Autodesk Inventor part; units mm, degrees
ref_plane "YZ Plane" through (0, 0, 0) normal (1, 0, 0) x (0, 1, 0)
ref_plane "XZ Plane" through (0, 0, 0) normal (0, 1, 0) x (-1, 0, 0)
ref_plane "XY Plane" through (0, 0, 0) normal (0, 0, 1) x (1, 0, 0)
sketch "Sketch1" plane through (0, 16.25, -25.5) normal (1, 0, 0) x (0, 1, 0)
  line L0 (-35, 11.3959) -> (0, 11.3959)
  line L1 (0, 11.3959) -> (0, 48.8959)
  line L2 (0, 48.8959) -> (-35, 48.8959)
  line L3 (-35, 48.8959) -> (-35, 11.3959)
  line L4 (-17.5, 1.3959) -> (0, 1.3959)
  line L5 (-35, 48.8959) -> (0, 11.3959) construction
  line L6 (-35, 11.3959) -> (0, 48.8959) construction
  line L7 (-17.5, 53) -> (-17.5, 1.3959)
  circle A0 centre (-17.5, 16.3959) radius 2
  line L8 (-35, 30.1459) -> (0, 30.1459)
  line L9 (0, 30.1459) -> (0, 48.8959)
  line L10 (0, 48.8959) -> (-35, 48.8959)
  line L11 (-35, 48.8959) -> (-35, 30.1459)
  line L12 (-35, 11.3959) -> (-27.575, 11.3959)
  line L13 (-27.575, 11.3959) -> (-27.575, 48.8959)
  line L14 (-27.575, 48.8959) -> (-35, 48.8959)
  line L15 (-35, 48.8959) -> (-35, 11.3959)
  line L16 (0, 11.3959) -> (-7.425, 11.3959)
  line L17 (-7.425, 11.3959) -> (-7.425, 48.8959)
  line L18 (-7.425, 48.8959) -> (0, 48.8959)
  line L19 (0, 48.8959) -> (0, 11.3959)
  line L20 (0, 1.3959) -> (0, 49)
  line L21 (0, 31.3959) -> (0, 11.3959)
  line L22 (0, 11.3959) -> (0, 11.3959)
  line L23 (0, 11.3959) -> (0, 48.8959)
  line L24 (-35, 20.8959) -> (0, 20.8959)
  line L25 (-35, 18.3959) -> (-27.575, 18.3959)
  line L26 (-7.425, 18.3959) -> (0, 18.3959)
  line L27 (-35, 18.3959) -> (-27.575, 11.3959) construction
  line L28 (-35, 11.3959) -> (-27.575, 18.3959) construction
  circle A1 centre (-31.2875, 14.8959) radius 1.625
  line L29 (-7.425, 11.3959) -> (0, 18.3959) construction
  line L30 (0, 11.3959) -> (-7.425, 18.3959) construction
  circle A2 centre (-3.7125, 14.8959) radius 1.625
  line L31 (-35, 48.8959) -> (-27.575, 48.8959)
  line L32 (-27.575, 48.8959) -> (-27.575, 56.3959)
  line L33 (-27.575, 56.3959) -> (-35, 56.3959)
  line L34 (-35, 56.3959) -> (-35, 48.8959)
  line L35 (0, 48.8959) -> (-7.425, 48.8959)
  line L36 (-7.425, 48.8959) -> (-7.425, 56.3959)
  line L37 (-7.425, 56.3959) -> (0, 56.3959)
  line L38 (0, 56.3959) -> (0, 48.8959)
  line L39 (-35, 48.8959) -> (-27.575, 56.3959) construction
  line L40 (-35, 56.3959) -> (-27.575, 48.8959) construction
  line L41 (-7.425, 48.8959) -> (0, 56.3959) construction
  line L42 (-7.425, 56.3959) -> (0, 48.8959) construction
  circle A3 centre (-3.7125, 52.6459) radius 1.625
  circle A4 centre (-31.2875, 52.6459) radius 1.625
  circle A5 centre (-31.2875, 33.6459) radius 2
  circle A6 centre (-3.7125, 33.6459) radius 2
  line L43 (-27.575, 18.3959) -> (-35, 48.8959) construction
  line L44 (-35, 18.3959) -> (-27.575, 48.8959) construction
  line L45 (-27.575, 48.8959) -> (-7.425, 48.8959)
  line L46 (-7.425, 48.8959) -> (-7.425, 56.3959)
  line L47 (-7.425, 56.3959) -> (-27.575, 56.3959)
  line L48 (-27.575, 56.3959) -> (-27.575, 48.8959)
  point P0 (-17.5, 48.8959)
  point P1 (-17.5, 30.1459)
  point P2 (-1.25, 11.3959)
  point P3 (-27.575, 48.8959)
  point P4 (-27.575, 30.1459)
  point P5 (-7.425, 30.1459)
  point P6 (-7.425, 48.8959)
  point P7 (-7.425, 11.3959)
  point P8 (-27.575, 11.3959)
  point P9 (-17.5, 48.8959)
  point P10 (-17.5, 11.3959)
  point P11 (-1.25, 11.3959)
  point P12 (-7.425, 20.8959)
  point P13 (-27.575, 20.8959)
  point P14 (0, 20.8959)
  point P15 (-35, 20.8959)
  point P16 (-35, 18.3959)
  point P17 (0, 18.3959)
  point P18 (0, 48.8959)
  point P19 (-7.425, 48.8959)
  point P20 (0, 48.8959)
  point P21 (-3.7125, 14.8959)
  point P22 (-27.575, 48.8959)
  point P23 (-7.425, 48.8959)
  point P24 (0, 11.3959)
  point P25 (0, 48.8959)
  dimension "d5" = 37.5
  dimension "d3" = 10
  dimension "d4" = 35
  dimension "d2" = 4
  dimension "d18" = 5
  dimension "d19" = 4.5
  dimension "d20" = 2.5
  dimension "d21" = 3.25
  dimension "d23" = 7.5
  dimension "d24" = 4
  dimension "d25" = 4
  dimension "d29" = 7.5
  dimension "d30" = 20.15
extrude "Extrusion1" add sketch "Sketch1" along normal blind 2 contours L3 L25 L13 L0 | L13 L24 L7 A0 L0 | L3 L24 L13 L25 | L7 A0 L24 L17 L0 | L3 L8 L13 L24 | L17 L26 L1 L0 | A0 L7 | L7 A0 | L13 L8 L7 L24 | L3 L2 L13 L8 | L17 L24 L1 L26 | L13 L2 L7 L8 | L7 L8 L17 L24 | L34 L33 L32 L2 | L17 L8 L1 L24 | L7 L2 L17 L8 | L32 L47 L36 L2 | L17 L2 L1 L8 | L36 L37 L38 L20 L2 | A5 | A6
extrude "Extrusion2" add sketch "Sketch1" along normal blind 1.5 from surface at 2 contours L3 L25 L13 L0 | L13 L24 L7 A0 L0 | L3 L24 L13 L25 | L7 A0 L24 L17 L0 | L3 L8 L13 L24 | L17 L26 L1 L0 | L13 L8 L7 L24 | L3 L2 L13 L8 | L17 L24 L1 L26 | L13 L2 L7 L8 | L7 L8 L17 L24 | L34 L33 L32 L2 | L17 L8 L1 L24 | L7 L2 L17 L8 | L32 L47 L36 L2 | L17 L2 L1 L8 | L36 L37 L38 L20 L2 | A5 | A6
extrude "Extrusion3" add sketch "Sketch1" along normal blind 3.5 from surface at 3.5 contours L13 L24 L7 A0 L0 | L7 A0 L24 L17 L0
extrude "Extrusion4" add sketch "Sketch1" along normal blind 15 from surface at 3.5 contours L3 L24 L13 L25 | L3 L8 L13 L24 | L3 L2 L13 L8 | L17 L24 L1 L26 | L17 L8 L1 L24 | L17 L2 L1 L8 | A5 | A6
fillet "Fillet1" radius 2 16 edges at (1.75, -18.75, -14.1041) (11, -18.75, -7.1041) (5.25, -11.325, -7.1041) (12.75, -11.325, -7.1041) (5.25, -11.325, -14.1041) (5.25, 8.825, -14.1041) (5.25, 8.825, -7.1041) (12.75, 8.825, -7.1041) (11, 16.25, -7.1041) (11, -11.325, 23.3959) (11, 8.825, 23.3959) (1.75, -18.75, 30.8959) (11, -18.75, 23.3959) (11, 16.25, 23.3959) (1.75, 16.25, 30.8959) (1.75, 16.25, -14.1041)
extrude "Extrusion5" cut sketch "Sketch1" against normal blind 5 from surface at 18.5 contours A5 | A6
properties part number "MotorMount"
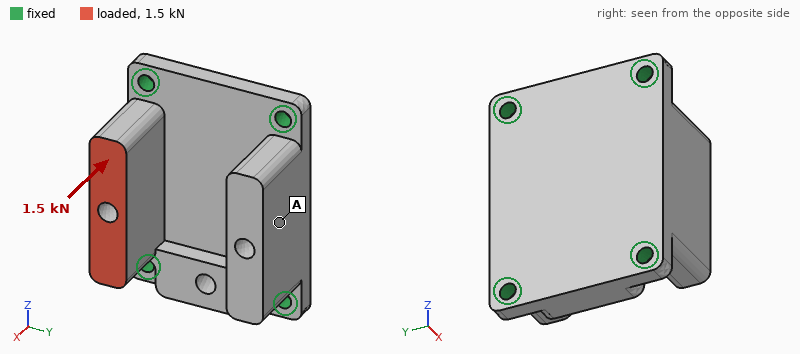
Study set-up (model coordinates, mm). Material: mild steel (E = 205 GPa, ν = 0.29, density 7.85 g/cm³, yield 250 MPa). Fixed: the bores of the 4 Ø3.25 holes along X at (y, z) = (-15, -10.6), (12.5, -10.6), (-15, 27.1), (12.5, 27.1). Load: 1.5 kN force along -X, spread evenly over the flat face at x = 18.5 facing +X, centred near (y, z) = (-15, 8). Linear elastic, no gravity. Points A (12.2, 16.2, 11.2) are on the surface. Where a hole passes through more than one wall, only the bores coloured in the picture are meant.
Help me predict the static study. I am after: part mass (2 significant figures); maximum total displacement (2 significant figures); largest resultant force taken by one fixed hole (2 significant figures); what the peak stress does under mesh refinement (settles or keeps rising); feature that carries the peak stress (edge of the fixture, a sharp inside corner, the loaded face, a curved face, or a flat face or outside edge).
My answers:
99 g
5.5 µm
830 N
keeps rising
edge of the fixture
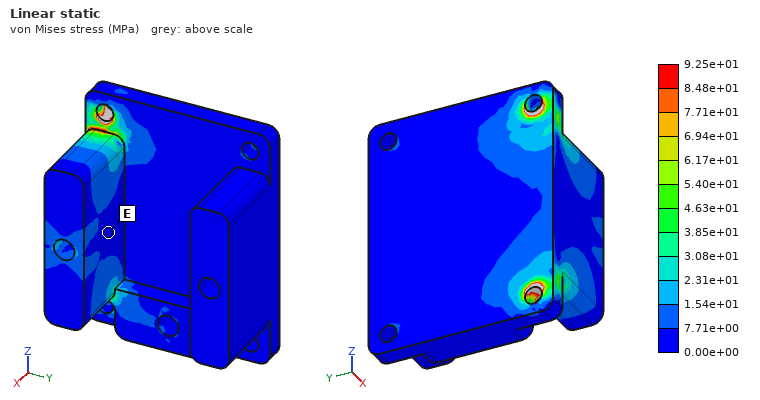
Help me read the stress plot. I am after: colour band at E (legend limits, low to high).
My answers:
0.00e+00 to 7.71e+00 MPa
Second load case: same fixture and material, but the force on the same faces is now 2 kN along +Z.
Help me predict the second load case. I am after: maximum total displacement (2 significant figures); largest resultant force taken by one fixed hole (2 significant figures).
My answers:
8.6 µm
1.4 kN
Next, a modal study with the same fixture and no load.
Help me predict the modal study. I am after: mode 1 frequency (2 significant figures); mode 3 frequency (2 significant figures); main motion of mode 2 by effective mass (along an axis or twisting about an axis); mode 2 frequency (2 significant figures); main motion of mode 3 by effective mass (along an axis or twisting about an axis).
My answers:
8300 Hz
16 kHz
along Y
9900 Hz
along X
